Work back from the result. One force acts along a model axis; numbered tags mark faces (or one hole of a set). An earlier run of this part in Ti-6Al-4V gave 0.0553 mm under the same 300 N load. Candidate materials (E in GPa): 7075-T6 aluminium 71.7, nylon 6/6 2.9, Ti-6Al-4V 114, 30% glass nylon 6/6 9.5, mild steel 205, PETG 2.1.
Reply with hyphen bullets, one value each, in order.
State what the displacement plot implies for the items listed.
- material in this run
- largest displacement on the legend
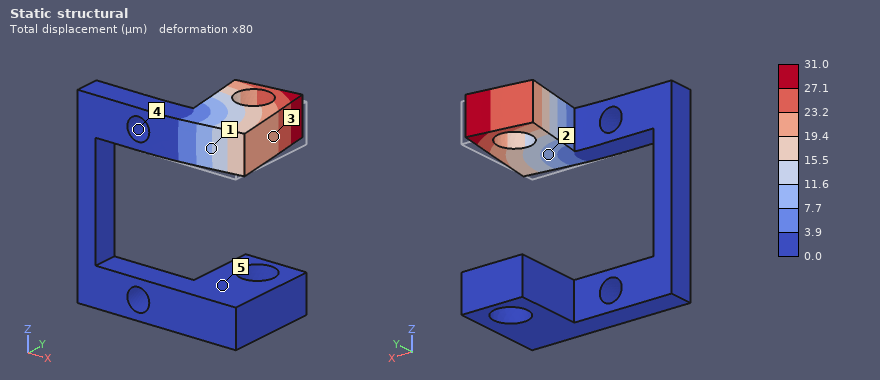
- mild steel
- 31.0 µm
